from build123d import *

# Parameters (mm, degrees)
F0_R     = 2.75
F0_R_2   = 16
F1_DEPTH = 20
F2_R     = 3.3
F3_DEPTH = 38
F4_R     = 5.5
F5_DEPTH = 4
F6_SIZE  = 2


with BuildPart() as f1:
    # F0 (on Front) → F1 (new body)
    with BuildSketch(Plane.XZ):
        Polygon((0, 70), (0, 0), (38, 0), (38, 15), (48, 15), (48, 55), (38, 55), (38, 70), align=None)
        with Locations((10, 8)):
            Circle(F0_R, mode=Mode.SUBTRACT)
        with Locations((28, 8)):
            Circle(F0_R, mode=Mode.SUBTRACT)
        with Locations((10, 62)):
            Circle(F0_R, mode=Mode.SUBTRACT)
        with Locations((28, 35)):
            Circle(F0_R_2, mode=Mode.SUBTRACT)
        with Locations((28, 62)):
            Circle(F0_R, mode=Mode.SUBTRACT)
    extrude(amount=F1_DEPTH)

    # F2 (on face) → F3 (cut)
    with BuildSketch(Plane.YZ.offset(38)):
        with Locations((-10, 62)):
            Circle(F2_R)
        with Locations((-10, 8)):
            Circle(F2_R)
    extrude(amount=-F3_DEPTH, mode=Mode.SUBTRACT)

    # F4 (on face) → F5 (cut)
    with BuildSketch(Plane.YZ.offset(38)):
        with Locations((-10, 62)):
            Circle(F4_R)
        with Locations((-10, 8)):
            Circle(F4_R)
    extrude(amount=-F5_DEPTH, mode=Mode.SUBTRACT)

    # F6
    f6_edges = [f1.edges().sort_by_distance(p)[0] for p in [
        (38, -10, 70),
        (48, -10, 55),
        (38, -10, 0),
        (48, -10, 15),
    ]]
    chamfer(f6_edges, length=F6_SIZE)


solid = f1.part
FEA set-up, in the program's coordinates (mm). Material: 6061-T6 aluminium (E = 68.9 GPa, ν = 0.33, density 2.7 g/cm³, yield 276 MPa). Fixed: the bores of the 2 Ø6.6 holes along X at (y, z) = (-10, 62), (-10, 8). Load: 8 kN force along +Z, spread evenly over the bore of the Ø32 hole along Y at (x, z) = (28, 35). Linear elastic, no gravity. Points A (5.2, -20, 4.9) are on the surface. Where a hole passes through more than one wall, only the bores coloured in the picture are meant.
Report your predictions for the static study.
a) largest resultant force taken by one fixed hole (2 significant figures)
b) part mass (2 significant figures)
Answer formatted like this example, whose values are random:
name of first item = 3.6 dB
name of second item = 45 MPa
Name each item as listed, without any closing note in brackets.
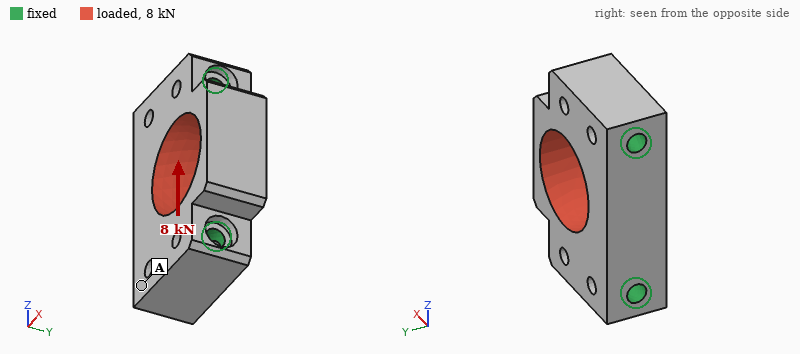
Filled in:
largest resultant force taken by one fixed hole = 4.0 kN
part mass = 110 g
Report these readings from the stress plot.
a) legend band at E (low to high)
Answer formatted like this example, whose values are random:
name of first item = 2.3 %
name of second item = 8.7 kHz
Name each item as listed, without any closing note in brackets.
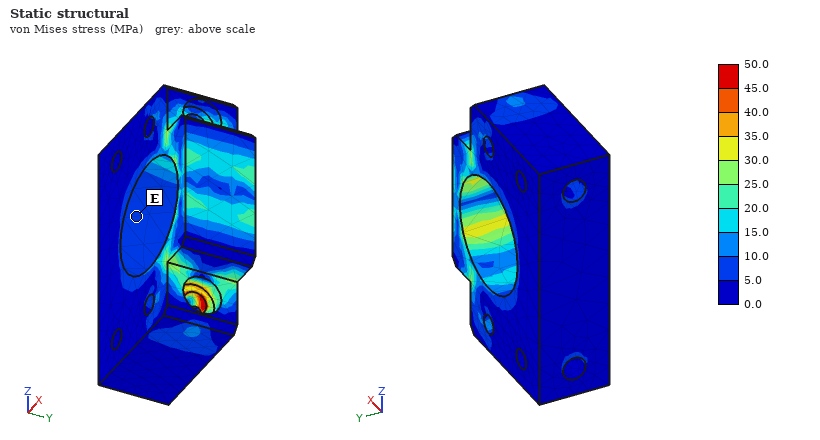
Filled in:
legend band at E = 5.0 to 10.0 MPa
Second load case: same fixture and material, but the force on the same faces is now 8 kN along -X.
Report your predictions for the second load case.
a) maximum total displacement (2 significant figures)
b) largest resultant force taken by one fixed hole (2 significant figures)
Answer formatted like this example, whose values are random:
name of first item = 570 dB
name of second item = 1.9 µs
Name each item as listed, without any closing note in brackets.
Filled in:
maximum total displacement = 13 µm
largest resultant force taken by one fixed hole = 4.1 kN
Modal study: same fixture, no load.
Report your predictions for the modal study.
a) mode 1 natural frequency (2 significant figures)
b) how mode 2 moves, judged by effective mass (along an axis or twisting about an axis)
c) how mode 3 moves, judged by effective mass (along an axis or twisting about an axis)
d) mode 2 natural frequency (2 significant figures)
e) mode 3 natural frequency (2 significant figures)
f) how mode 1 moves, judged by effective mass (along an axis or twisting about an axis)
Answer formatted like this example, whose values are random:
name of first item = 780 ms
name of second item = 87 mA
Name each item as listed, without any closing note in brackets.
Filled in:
mode 1 natural frequency = 14 kHz
how mode 2 moves, judged by effective mass = along Z
how mode 3 moves, judged by effective mass = along Y
mode 2 natural frequency = 19 kHz
mode 3 natural frequency = 21 kHz
how mode 1 moves, judged by effective mass = along Y
